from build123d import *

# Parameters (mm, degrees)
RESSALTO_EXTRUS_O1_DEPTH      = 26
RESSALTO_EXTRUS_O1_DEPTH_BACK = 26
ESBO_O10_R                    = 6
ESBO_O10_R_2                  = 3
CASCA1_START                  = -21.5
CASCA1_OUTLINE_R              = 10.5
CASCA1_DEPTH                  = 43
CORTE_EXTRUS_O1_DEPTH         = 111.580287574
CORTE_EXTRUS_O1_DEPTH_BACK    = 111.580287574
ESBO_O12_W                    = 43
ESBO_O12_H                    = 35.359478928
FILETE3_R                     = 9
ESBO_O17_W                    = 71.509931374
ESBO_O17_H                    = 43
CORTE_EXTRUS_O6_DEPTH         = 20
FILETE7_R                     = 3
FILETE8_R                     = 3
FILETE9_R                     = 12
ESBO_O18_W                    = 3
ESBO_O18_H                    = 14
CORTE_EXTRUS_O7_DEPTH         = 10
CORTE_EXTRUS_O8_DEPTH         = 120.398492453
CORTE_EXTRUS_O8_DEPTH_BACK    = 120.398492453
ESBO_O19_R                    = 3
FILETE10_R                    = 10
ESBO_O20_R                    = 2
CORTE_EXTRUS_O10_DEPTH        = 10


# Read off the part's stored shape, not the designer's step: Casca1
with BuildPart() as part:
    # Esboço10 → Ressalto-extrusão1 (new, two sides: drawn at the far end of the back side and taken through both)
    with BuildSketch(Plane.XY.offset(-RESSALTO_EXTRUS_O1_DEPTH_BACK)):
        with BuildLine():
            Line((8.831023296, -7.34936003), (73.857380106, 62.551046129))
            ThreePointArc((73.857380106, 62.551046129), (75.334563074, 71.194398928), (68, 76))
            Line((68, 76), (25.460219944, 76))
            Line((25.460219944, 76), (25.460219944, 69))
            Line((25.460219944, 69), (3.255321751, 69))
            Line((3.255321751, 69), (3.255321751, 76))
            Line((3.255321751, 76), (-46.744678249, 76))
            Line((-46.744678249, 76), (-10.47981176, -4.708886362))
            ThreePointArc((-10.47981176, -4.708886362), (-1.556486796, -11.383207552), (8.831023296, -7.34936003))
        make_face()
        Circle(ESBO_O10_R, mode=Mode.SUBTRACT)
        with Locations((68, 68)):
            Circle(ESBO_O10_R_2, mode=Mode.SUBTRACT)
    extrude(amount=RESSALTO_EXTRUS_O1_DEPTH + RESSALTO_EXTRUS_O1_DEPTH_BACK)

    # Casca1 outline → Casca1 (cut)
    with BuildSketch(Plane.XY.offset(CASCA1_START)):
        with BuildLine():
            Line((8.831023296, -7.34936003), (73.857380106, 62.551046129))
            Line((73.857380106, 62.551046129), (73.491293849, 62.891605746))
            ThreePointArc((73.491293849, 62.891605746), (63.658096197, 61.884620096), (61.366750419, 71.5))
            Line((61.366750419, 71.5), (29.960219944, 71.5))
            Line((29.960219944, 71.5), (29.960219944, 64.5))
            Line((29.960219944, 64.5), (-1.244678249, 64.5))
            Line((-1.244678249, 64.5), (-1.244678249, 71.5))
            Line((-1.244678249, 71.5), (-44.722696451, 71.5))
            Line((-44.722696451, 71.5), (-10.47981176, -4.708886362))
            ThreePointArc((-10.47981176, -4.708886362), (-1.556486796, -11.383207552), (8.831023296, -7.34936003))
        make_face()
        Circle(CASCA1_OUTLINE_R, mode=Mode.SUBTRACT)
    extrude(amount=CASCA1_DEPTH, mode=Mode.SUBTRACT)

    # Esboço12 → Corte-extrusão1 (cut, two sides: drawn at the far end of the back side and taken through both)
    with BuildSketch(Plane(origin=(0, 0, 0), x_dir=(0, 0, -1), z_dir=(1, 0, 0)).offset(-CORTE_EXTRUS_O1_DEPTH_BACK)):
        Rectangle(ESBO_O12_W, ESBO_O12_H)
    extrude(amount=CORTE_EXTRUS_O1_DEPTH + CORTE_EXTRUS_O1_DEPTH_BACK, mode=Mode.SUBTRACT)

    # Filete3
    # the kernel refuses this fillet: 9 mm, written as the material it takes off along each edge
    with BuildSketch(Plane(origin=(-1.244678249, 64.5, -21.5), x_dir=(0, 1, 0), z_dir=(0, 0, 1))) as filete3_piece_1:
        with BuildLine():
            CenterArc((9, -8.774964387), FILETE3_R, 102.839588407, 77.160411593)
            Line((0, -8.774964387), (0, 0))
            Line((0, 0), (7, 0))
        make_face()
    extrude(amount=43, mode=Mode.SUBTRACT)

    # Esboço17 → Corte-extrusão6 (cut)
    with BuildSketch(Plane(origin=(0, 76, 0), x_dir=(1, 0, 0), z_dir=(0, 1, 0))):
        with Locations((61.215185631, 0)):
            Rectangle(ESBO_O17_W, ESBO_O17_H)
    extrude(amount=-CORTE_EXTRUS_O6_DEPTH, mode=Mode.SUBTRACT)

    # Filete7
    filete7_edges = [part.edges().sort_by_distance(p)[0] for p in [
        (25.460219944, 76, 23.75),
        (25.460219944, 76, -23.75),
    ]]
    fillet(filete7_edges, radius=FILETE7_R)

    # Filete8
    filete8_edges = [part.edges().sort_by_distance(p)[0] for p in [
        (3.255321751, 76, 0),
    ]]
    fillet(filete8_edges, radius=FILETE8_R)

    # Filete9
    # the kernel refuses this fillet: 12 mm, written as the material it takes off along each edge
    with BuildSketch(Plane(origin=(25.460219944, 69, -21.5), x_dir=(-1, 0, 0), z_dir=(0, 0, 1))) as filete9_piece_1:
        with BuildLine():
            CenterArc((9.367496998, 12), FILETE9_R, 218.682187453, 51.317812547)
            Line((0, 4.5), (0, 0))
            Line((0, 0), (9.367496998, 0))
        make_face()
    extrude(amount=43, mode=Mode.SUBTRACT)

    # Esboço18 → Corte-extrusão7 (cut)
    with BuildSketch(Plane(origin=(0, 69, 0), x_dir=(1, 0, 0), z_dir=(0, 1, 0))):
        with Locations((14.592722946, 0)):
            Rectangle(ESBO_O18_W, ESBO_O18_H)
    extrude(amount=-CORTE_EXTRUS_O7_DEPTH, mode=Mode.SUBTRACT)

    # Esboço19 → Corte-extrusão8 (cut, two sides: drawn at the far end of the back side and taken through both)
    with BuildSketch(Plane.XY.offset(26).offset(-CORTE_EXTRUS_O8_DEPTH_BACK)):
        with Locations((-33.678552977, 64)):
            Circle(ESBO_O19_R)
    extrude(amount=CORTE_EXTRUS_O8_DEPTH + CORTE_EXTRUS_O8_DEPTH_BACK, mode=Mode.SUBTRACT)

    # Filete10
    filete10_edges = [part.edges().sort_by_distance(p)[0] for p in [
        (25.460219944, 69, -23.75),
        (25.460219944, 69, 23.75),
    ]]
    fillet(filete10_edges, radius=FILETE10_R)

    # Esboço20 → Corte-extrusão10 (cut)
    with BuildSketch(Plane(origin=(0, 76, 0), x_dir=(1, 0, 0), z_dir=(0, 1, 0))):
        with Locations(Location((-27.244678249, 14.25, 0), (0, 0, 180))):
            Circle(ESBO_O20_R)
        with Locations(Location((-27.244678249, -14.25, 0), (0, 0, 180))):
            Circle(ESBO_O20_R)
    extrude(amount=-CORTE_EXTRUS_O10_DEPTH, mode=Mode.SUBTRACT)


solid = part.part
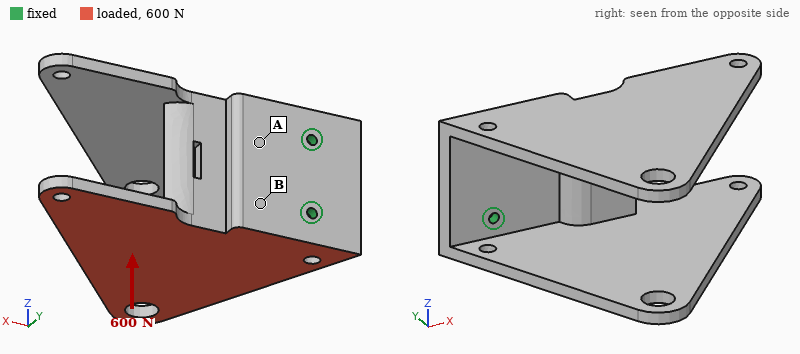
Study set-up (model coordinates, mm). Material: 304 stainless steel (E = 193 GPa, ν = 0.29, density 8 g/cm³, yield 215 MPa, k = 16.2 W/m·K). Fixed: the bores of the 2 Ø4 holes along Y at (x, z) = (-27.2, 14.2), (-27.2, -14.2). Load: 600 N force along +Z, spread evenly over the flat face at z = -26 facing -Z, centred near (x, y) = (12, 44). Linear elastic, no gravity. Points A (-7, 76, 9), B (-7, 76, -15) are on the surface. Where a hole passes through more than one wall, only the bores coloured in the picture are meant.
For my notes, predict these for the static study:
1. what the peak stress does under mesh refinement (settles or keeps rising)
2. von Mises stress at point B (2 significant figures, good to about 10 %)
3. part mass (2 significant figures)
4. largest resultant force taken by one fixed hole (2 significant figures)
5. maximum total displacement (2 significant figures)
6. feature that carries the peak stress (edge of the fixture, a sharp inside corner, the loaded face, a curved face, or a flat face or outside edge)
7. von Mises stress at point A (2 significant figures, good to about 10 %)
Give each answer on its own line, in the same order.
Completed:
keeps rising
35 MPa
540 g
940 N
0.40 mm
edge of the fixture
12 MPa
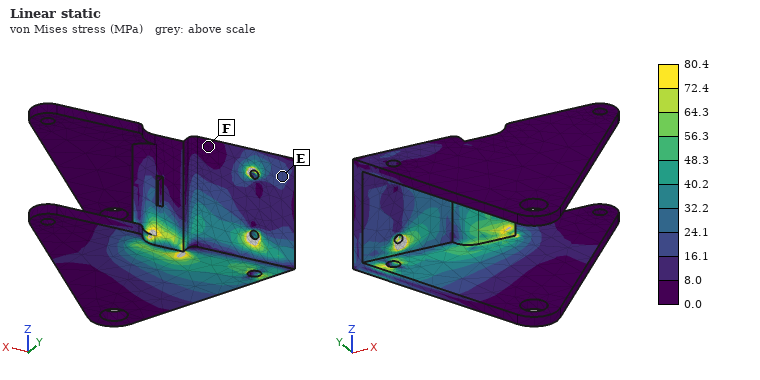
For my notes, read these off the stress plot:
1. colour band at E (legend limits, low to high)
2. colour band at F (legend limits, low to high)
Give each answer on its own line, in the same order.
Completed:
16.1 to 24.1 MPa
0.0 to 8.0 MPa
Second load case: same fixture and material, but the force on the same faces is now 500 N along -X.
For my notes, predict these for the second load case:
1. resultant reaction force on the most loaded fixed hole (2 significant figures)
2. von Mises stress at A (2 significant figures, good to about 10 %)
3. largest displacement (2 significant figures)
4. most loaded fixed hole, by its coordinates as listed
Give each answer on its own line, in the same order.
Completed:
670 N
17 MPa
0.15 mm
(-27.2, -14.2)
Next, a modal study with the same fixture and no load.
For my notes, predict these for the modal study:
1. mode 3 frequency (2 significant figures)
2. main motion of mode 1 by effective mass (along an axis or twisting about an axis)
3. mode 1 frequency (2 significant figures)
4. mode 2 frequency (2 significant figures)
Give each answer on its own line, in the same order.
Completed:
630 Hz
along Z
470 Hz
500 Hz
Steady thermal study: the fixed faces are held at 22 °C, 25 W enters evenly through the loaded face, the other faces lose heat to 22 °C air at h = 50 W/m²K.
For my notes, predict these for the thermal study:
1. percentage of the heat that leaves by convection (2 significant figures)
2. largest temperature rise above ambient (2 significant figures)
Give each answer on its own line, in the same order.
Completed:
86 %
57 K
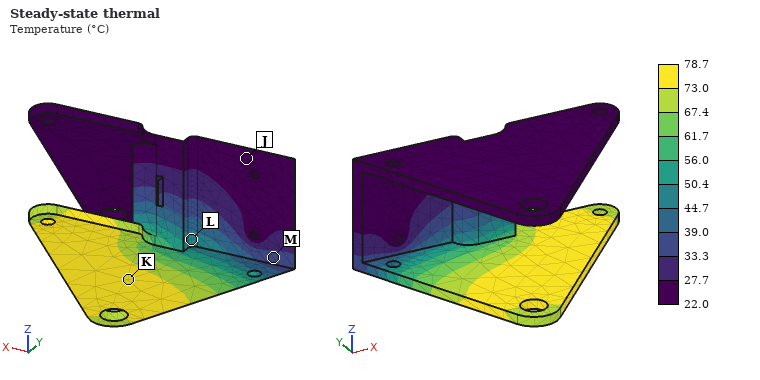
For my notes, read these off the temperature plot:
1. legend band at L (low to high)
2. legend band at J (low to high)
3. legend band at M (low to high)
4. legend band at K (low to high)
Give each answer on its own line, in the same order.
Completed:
44.7 to 50.4 °C
22.0 to 27.7 °C
33.3 to 39.0 °C
73.0 to 78.7 °C
